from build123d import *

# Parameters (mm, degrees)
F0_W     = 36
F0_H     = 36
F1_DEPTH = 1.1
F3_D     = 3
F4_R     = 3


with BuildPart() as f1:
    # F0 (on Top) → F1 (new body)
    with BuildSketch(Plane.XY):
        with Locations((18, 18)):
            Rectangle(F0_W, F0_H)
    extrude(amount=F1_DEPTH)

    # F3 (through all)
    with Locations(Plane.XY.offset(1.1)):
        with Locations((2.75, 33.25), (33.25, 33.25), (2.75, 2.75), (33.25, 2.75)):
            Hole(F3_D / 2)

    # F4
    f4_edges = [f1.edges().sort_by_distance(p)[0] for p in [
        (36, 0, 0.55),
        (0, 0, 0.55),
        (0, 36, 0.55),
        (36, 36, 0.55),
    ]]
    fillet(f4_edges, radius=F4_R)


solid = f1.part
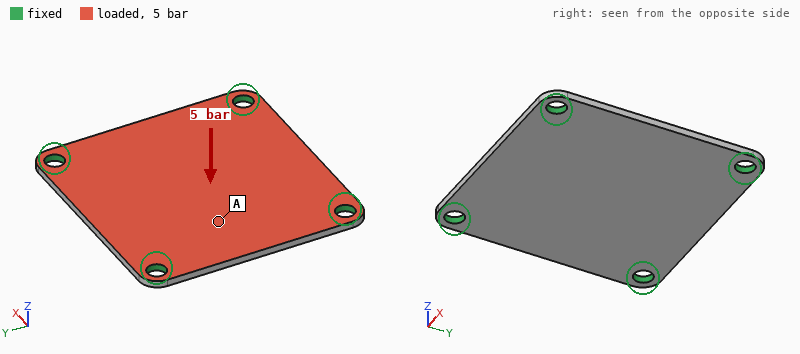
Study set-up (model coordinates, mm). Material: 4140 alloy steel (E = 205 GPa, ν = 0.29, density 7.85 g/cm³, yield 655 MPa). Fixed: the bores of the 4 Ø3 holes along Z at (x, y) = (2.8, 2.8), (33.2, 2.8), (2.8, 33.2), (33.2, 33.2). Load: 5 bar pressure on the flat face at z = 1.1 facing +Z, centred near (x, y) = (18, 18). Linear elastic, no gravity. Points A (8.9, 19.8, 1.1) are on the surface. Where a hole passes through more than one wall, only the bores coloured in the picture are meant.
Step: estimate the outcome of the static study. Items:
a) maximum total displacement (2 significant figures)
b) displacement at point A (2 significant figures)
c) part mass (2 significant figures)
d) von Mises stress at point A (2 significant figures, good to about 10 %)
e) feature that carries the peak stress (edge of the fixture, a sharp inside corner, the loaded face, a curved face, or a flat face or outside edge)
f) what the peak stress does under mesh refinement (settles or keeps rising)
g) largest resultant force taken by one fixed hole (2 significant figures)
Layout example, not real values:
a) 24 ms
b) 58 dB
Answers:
a) 0.11 mm
b) 0.082 mm
c) 11 g
d) 97 MPa
e) edge of the fixture
f) keeps rising
g) 160 N
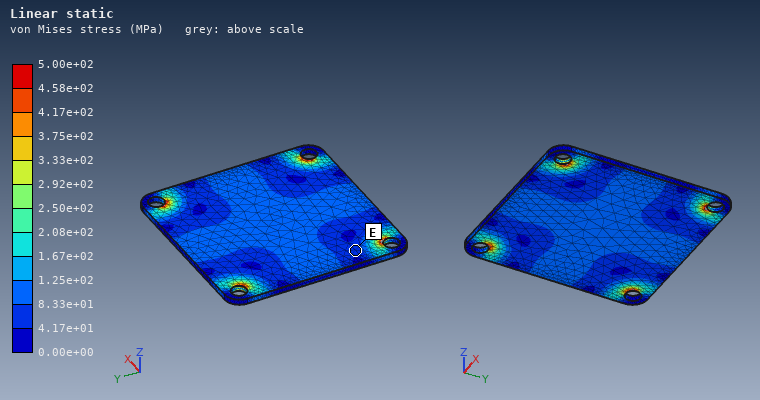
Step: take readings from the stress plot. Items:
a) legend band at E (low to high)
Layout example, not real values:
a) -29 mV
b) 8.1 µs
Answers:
a) 4.17e+01 to 8.33e+01 MPa
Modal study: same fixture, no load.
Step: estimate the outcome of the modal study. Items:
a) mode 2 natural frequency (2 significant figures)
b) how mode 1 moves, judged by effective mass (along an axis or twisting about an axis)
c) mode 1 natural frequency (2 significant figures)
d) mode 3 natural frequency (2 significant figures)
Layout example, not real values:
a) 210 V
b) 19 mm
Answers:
a) 7700 Hz
b) along Z
c) 4500 Hz
d) 7700 Hz
